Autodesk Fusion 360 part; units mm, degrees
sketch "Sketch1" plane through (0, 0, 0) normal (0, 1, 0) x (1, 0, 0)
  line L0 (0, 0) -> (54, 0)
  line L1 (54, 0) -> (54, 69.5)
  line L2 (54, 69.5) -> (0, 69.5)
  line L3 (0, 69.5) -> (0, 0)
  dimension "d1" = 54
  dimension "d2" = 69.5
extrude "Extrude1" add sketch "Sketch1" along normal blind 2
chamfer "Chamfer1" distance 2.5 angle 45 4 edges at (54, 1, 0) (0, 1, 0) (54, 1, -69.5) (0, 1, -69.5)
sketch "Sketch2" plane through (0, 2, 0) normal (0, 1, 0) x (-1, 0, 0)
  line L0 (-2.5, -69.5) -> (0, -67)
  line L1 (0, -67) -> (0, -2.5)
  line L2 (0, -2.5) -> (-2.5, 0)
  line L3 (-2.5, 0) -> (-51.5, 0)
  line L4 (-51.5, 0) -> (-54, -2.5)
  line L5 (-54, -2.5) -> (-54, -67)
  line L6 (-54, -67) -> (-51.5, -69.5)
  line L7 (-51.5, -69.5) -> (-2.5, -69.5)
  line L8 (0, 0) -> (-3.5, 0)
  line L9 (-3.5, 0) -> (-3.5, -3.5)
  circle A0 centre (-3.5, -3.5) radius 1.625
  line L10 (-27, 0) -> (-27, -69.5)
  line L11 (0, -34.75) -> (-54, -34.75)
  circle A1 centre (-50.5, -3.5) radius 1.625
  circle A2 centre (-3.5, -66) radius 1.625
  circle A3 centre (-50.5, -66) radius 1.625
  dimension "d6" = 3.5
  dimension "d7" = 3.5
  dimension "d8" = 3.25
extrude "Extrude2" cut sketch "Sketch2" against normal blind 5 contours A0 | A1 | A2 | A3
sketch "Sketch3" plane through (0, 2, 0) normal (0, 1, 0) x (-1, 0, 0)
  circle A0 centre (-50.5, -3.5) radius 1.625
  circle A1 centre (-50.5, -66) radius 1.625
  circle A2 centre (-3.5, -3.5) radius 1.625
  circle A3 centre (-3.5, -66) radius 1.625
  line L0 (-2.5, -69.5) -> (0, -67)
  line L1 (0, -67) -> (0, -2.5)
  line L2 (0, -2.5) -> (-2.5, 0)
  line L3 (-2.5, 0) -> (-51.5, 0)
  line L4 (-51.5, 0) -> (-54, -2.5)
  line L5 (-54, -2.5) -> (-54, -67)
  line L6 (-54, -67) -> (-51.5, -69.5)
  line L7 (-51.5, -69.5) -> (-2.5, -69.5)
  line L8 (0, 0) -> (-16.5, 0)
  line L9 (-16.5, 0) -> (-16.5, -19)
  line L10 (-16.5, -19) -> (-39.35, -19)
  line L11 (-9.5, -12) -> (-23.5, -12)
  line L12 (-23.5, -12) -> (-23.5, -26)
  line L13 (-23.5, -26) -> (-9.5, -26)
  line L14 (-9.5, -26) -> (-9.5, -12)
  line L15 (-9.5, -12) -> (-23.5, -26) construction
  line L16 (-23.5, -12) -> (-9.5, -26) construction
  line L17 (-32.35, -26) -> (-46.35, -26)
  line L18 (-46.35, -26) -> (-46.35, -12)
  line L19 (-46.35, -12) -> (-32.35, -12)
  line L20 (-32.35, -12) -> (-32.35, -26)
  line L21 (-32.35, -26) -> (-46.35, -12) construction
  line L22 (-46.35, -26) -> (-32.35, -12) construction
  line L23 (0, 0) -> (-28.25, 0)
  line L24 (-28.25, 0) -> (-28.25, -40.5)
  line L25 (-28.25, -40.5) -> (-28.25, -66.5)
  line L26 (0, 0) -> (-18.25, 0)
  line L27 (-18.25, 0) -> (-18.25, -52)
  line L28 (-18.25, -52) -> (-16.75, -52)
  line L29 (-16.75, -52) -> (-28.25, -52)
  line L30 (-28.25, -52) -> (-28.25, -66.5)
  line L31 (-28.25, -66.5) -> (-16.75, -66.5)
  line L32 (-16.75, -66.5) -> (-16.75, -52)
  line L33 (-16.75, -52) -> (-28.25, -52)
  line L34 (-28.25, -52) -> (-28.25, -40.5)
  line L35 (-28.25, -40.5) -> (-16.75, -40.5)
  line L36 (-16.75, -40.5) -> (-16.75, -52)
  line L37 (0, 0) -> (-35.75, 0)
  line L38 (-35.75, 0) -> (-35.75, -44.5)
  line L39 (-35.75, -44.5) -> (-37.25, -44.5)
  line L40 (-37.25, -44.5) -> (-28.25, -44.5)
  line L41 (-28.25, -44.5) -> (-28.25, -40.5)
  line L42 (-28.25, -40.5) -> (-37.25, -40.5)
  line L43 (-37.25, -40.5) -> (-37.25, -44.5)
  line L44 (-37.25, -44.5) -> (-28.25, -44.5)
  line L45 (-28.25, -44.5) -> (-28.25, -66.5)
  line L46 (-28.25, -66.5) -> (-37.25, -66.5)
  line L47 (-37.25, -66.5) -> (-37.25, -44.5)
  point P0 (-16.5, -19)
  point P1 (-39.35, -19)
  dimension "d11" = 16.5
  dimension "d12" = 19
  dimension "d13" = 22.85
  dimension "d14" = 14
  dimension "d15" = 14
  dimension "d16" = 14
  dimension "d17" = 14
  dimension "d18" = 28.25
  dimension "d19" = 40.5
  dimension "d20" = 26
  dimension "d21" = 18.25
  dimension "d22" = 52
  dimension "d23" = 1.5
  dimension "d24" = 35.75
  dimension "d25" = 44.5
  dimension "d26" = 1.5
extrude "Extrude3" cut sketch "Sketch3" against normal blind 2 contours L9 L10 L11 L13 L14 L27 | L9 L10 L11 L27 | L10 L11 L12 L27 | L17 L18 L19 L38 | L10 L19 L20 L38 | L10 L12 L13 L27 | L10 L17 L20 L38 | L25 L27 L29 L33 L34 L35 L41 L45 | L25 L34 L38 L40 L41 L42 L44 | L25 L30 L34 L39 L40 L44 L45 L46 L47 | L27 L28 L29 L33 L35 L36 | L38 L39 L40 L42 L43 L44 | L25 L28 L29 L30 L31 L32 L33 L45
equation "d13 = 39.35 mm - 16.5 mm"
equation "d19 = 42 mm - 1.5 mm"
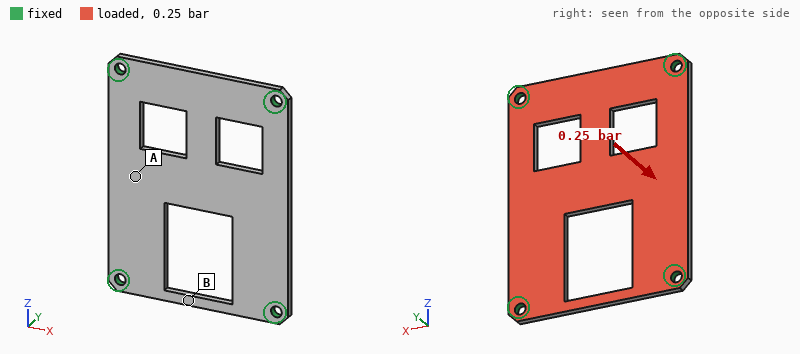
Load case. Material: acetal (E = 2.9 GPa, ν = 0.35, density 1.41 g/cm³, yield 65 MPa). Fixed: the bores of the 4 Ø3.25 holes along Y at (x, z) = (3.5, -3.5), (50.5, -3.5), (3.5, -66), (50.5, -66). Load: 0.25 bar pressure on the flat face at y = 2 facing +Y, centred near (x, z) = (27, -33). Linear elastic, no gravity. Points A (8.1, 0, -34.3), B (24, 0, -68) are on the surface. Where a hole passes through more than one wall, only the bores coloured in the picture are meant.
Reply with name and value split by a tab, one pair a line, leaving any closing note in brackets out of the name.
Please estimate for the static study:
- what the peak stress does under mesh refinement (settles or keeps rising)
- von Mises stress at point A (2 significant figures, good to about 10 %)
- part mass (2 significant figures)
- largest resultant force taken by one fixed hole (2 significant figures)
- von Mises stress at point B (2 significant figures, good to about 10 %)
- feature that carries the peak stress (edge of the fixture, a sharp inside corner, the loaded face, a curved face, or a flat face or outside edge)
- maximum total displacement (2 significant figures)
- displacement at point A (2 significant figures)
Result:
what the peak stress does under mesh refinement	keeps rising
von Mises stress at point A	6.2 MPa
part mass	7.8 g
largest resultant force taken by one fixed hole	18 N
von Mises stress at point B	2.9 MPa
feature that carries the peak stress	edge of the fixture
maximum total displacement	0.90 mm
displacement at point A	0.69 mm
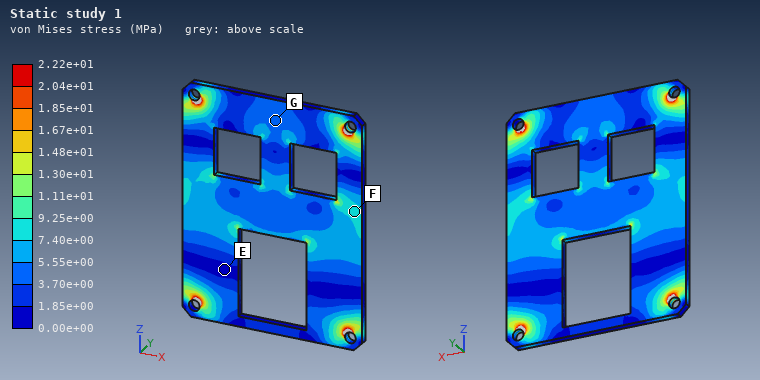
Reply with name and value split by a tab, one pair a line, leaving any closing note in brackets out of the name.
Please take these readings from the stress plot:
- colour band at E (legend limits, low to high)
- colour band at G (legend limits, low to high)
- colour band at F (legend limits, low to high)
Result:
colour band at E	0.00e+00 to 1.85e+00 MPa
colour band at G	3.70e+00 to 5.55e+00 MPa
colour band at F	7.40e+00 to 9.25e+00 MPa
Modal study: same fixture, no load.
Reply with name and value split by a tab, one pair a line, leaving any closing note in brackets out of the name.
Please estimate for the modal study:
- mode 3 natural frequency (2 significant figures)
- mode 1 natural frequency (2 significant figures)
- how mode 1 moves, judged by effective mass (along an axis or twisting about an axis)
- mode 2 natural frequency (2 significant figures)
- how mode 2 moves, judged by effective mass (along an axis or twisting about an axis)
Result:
mode 3 natural frequency	1300 Hz
mode 1 natural frequency	600 Hz
how mode 1 moves, judged by effective mass	along Y
mode 2 natural frequency	870 Hz
how mode 2 moves, judged by effective mass	twisting about Z
